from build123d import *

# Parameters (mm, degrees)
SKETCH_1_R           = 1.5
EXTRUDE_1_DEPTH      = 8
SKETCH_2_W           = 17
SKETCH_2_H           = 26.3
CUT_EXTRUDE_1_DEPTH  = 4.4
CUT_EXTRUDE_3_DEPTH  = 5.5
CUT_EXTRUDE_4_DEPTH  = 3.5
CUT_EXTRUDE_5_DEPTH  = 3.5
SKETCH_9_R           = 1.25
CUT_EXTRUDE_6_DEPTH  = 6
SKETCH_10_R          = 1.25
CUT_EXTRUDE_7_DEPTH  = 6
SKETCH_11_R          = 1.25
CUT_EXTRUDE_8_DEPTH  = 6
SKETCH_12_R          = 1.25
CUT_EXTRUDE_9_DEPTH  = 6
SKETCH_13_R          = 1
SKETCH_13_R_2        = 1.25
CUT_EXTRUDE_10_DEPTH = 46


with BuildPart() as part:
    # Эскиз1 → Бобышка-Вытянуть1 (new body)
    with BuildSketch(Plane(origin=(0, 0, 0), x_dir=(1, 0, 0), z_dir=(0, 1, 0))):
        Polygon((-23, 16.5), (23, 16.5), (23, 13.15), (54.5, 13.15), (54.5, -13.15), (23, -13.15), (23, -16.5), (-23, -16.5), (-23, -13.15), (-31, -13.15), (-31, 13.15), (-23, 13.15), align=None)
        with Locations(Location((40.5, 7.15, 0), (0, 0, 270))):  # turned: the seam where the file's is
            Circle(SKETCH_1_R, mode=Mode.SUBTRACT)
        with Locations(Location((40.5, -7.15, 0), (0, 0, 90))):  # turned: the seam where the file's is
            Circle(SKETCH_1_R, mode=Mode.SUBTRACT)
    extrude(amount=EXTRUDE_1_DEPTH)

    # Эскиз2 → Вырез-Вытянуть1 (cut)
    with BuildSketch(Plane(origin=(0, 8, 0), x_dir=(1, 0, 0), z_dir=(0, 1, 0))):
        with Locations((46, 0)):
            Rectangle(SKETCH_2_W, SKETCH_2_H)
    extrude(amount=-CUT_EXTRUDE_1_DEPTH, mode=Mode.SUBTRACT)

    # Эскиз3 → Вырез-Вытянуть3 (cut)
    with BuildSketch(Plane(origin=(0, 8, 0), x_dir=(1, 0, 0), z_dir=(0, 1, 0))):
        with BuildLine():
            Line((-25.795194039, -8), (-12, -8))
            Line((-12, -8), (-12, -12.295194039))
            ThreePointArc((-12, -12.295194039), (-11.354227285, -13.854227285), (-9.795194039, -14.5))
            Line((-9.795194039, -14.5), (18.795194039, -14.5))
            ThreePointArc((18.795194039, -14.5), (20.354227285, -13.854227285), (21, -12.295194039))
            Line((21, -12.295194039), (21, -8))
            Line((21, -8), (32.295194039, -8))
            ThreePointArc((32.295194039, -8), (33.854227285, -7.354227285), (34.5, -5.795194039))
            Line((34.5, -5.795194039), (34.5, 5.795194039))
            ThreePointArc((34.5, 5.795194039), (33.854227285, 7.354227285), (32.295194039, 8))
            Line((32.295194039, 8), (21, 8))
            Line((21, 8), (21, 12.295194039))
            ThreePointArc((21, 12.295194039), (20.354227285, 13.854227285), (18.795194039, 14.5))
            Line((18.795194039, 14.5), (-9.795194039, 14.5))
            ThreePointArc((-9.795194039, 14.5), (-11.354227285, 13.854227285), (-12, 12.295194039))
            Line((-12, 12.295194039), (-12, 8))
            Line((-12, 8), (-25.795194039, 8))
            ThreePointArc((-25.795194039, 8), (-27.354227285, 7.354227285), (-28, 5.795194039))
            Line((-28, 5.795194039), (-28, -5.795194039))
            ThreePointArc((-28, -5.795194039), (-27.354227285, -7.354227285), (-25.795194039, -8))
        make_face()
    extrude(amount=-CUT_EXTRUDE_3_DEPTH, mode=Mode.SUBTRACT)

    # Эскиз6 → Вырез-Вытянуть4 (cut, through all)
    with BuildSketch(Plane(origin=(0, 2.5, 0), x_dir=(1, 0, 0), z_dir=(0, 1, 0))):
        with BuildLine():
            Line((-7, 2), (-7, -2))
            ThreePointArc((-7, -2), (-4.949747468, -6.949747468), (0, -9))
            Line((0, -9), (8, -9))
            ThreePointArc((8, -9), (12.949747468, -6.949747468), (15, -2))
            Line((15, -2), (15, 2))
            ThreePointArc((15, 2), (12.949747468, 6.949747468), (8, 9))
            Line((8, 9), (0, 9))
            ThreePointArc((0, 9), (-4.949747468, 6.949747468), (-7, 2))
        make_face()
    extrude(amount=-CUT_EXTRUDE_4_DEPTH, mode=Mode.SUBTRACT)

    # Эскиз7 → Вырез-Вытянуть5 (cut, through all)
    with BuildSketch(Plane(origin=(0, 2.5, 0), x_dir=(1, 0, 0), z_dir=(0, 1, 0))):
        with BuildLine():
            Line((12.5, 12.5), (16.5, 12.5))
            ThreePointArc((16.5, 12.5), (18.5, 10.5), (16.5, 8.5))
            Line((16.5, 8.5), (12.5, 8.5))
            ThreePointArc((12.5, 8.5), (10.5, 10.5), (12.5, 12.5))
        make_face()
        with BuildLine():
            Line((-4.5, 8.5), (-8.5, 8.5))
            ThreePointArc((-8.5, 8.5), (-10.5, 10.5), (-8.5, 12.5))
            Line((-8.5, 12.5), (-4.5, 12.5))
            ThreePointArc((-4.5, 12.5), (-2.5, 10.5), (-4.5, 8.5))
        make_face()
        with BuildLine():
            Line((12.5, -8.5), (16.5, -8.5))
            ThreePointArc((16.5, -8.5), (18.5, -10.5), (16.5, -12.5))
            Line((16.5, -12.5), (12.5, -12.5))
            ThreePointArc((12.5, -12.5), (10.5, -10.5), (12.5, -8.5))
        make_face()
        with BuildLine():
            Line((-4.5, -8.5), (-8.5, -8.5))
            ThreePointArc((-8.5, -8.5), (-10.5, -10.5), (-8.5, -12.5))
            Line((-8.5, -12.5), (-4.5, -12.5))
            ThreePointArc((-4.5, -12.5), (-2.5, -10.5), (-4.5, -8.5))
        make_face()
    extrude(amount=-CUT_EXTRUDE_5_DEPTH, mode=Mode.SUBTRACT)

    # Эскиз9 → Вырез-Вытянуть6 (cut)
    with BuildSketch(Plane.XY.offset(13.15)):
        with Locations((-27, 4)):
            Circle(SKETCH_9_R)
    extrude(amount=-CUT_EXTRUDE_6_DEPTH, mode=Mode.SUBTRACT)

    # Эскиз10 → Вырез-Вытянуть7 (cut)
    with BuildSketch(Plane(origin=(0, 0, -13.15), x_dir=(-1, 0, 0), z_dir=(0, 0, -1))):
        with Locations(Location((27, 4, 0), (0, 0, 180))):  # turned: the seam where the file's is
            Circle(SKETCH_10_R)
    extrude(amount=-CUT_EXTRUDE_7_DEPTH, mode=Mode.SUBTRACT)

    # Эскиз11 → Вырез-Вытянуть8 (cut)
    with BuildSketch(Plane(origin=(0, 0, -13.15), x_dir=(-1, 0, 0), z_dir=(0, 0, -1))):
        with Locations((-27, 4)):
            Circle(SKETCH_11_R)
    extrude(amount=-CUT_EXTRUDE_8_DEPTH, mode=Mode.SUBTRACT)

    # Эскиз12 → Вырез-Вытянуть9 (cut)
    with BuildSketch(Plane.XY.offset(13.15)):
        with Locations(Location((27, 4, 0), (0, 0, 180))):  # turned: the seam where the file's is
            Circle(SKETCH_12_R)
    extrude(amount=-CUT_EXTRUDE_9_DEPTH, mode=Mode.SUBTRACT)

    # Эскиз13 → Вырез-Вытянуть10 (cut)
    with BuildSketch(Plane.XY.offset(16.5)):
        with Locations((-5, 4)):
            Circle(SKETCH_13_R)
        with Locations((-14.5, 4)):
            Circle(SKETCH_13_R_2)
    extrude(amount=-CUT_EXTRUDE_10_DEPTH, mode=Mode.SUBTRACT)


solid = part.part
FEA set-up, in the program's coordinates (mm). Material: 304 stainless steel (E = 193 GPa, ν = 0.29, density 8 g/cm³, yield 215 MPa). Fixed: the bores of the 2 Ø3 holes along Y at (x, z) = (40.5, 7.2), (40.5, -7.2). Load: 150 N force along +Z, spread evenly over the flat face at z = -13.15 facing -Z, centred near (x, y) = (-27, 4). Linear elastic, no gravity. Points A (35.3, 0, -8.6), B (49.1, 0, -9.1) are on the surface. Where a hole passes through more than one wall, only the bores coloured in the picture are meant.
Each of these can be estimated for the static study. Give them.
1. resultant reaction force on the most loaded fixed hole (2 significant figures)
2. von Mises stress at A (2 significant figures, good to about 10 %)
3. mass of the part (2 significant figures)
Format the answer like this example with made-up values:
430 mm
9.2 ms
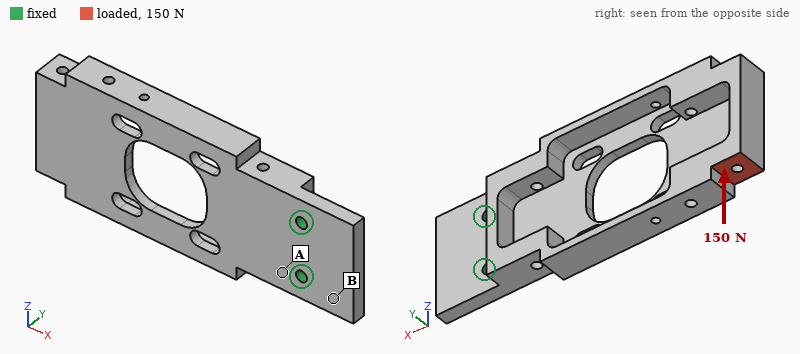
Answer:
640 N
20 MPa
74 g
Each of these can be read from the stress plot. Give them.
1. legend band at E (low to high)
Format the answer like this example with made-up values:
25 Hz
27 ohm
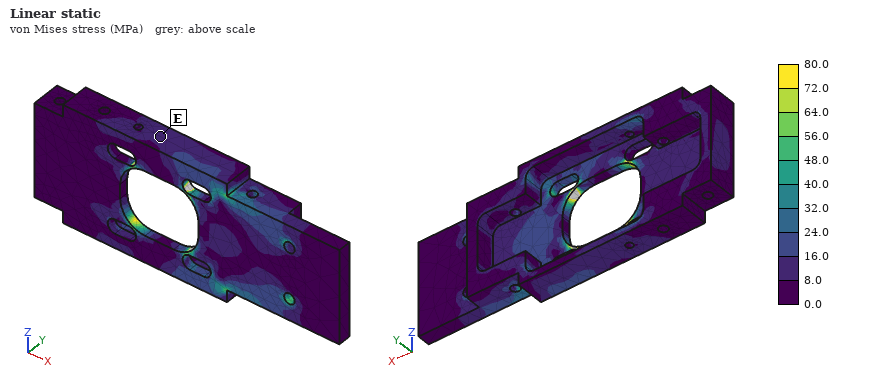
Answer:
8.0 to 16.0 MPa
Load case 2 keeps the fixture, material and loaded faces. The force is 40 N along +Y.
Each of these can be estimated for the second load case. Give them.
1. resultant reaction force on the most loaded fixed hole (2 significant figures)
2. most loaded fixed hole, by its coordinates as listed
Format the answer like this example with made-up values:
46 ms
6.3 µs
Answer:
59 N
(40.5, -7.2)
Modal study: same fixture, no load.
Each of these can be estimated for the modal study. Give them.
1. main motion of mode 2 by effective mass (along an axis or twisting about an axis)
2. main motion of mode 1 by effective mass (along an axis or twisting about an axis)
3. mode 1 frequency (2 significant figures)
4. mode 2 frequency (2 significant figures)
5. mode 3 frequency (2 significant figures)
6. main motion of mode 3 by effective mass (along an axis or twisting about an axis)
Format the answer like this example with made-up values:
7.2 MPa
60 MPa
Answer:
along Z
along Y
660 Hz
1800 Hz
2600 Hz
along Z
